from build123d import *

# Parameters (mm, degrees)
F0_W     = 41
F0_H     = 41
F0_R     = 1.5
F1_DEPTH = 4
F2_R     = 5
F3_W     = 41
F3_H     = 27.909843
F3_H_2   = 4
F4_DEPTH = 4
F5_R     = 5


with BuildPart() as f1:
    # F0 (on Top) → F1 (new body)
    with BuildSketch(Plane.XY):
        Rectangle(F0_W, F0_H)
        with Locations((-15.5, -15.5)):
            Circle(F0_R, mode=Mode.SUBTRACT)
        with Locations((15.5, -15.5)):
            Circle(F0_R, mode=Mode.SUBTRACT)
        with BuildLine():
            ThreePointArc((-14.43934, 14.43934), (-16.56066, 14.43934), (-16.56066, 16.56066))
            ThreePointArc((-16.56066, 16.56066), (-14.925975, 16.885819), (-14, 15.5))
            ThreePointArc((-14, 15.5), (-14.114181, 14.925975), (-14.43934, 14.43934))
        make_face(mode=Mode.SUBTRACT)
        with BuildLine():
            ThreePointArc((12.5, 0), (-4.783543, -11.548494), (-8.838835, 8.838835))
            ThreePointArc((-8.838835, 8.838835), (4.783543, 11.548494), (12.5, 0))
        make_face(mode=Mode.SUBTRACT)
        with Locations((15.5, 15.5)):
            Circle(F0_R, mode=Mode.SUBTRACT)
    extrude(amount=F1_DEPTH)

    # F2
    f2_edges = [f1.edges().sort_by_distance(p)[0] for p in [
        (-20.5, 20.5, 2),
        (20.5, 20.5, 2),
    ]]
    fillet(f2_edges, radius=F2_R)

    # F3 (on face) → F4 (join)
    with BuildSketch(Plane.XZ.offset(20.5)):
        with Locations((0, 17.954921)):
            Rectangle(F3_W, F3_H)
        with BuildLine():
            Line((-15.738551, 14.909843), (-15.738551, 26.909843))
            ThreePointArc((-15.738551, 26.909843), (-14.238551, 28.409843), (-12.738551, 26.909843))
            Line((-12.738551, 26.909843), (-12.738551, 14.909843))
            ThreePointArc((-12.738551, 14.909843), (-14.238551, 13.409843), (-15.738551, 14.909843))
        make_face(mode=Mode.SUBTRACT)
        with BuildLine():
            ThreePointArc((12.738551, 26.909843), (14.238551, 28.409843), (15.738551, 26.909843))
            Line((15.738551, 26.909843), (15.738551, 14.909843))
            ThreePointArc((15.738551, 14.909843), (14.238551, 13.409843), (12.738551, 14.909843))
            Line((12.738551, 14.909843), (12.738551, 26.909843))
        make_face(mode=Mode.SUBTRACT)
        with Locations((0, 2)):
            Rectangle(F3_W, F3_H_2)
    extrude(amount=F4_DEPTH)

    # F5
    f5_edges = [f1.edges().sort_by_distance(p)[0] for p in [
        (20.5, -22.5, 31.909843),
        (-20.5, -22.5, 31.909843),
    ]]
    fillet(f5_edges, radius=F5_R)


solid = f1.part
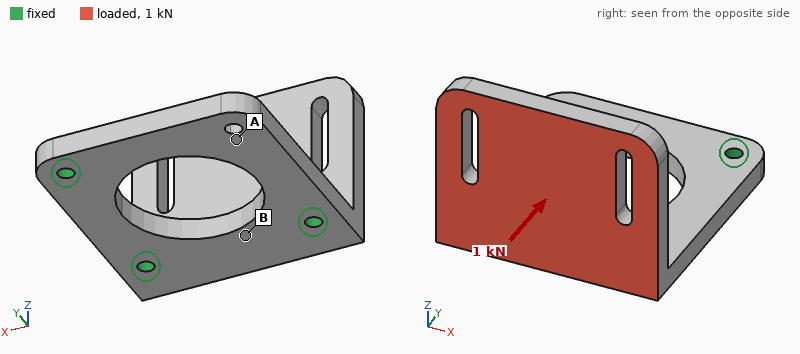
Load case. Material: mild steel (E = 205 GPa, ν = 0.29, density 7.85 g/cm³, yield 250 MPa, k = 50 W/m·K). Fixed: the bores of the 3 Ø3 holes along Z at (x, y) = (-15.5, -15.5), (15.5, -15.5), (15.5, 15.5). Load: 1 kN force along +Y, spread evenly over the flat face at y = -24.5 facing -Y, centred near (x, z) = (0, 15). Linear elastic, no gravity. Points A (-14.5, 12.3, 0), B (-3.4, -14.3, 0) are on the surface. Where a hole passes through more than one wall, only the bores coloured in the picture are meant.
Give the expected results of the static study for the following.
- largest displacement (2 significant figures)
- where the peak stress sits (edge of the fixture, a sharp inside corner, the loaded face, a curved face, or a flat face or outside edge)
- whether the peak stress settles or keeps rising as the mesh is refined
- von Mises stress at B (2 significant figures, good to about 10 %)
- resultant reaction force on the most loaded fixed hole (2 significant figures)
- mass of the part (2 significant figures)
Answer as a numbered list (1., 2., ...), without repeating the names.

1. 0.14 mm
2. edge of the fixture
3. keeps rising
4. 49 MPa
5. 530 N
6. 74 g
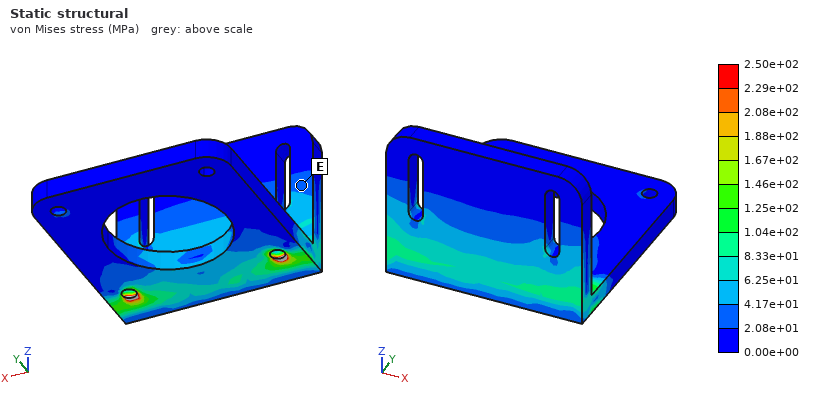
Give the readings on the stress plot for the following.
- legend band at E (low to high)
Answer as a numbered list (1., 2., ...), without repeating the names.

1. 2.08e+01 to 4.17e+01 MPa
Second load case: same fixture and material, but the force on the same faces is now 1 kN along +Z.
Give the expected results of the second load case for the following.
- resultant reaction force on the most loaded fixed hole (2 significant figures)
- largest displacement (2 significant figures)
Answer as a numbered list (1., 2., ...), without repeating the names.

1. 520 N
2. 47 µm
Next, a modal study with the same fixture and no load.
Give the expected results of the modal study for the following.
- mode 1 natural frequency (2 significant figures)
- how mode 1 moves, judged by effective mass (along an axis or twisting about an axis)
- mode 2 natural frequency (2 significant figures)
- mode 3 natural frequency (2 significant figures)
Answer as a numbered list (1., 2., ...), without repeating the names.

1. 2700 Hz
2. along Y
3. 4400 Hz
4. 6300 Hz
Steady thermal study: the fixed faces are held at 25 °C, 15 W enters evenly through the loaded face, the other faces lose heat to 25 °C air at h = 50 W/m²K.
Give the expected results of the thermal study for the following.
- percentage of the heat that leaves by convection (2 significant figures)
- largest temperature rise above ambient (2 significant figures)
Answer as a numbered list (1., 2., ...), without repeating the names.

1. 20 %
2. 35 K
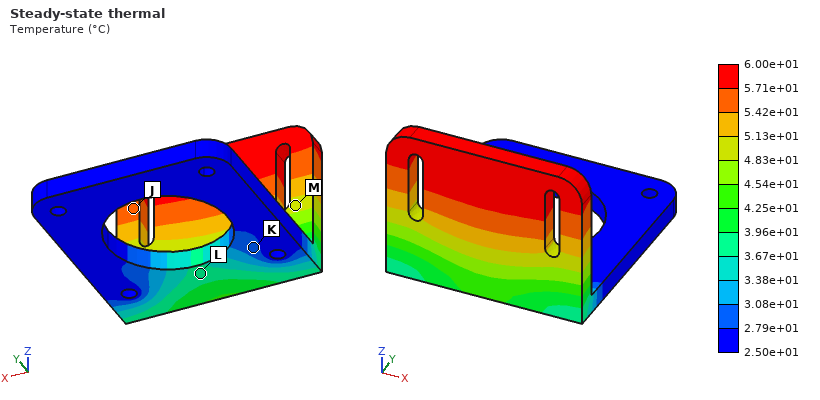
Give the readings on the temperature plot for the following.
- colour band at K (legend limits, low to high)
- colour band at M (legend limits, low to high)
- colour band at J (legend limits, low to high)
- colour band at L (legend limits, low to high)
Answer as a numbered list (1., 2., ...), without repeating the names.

1. 2.79e+01 to 3.08e+01 °C
2. 4.83e+01 to 5.13e+01 °C
3. 5.42e+01 to 5.71e+01 °C
4. 3.67e+01 to 3.96e+01 °C
